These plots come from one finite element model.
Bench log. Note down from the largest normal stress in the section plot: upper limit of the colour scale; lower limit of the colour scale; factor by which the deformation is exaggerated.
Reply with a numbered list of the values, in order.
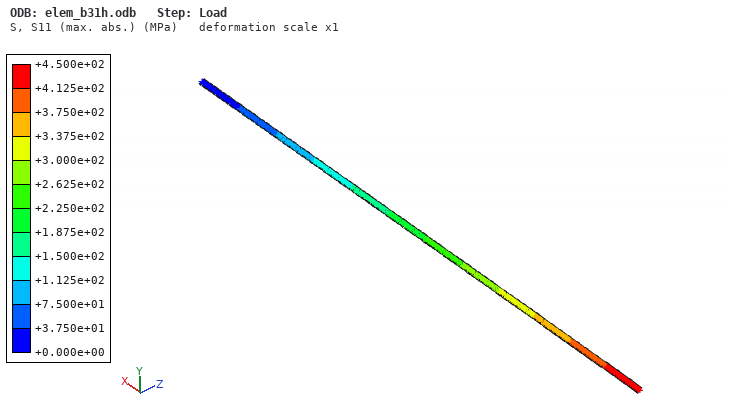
1. +4.500e+02 MPa
2. +0.000e+00 MPa
3. 1
